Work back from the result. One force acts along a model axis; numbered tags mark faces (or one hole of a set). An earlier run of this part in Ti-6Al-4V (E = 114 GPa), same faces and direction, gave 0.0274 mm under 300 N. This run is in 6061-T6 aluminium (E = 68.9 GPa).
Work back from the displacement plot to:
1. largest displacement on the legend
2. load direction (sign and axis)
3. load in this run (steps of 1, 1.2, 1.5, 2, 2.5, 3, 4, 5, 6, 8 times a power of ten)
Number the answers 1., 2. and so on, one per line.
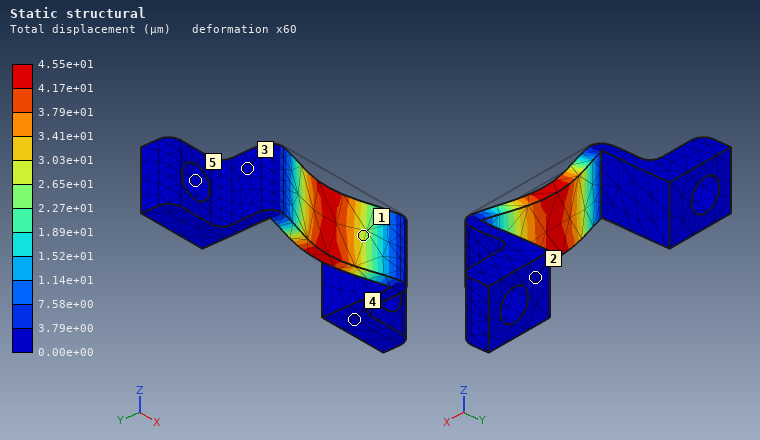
1. 4.55e+01 µm
2. +Y
3. 300 N
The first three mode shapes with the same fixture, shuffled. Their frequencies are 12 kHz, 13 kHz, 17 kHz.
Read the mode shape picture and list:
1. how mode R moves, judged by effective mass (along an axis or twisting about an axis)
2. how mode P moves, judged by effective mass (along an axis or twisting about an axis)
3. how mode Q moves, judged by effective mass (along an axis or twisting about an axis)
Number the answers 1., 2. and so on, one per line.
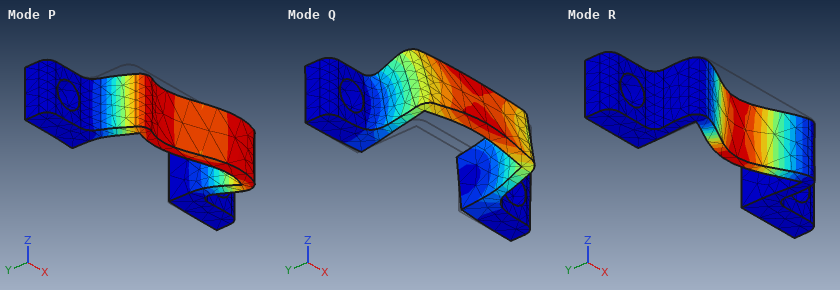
1. along Y
2. along X
3. along Z
